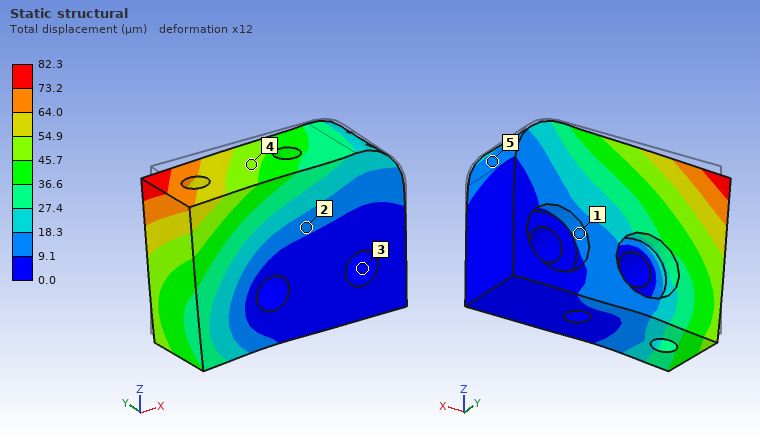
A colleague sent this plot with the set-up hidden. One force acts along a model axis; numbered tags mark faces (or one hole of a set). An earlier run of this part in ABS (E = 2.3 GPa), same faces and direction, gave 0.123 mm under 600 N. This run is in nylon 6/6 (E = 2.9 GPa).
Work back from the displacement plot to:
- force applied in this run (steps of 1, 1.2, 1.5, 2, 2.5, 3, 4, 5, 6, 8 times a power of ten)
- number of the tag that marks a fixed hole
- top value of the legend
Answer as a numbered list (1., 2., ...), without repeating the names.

1. 500 N
2. 3
3. 82.3 µm
